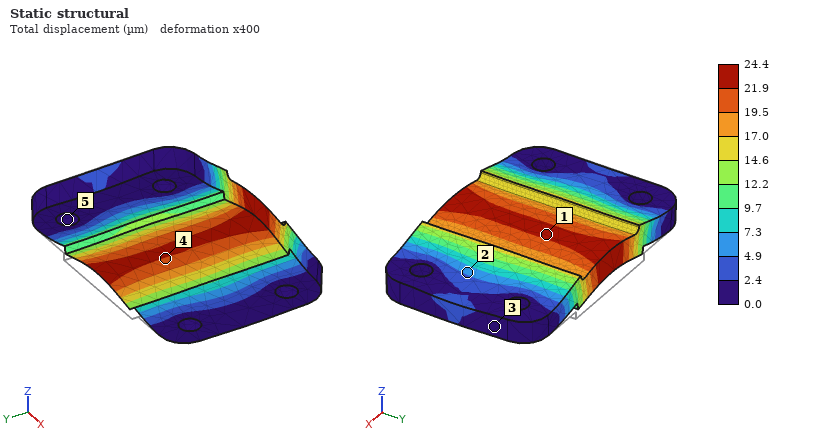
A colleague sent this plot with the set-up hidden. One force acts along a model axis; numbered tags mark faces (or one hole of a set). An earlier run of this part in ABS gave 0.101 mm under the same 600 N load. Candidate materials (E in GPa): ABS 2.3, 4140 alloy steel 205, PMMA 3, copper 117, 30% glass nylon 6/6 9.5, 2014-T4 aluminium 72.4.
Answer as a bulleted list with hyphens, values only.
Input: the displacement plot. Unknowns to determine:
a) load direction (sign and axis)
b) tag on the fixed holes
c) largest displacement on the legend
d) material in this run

- +Z
- 5
- 24.4 µm
- 30% glass nylon 6/6
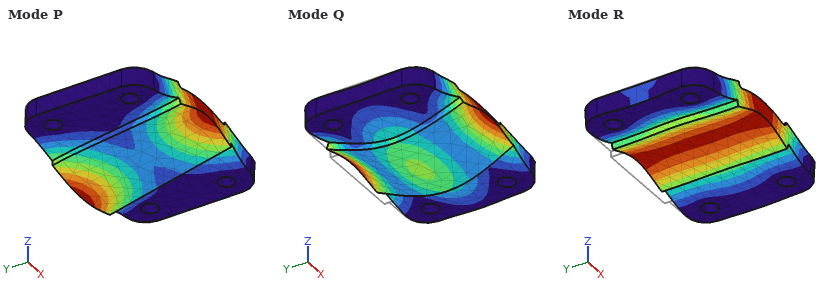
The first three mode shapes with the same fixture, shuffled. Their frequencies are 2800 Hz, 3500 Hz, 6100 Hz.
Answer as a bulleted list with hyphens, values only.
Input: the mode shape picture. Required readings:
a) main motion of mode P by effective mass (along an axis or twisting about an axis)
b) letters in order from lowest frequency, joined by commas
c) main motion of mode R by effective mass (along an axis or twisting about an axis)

- twisting about X
- R, P, Q
- along Z
